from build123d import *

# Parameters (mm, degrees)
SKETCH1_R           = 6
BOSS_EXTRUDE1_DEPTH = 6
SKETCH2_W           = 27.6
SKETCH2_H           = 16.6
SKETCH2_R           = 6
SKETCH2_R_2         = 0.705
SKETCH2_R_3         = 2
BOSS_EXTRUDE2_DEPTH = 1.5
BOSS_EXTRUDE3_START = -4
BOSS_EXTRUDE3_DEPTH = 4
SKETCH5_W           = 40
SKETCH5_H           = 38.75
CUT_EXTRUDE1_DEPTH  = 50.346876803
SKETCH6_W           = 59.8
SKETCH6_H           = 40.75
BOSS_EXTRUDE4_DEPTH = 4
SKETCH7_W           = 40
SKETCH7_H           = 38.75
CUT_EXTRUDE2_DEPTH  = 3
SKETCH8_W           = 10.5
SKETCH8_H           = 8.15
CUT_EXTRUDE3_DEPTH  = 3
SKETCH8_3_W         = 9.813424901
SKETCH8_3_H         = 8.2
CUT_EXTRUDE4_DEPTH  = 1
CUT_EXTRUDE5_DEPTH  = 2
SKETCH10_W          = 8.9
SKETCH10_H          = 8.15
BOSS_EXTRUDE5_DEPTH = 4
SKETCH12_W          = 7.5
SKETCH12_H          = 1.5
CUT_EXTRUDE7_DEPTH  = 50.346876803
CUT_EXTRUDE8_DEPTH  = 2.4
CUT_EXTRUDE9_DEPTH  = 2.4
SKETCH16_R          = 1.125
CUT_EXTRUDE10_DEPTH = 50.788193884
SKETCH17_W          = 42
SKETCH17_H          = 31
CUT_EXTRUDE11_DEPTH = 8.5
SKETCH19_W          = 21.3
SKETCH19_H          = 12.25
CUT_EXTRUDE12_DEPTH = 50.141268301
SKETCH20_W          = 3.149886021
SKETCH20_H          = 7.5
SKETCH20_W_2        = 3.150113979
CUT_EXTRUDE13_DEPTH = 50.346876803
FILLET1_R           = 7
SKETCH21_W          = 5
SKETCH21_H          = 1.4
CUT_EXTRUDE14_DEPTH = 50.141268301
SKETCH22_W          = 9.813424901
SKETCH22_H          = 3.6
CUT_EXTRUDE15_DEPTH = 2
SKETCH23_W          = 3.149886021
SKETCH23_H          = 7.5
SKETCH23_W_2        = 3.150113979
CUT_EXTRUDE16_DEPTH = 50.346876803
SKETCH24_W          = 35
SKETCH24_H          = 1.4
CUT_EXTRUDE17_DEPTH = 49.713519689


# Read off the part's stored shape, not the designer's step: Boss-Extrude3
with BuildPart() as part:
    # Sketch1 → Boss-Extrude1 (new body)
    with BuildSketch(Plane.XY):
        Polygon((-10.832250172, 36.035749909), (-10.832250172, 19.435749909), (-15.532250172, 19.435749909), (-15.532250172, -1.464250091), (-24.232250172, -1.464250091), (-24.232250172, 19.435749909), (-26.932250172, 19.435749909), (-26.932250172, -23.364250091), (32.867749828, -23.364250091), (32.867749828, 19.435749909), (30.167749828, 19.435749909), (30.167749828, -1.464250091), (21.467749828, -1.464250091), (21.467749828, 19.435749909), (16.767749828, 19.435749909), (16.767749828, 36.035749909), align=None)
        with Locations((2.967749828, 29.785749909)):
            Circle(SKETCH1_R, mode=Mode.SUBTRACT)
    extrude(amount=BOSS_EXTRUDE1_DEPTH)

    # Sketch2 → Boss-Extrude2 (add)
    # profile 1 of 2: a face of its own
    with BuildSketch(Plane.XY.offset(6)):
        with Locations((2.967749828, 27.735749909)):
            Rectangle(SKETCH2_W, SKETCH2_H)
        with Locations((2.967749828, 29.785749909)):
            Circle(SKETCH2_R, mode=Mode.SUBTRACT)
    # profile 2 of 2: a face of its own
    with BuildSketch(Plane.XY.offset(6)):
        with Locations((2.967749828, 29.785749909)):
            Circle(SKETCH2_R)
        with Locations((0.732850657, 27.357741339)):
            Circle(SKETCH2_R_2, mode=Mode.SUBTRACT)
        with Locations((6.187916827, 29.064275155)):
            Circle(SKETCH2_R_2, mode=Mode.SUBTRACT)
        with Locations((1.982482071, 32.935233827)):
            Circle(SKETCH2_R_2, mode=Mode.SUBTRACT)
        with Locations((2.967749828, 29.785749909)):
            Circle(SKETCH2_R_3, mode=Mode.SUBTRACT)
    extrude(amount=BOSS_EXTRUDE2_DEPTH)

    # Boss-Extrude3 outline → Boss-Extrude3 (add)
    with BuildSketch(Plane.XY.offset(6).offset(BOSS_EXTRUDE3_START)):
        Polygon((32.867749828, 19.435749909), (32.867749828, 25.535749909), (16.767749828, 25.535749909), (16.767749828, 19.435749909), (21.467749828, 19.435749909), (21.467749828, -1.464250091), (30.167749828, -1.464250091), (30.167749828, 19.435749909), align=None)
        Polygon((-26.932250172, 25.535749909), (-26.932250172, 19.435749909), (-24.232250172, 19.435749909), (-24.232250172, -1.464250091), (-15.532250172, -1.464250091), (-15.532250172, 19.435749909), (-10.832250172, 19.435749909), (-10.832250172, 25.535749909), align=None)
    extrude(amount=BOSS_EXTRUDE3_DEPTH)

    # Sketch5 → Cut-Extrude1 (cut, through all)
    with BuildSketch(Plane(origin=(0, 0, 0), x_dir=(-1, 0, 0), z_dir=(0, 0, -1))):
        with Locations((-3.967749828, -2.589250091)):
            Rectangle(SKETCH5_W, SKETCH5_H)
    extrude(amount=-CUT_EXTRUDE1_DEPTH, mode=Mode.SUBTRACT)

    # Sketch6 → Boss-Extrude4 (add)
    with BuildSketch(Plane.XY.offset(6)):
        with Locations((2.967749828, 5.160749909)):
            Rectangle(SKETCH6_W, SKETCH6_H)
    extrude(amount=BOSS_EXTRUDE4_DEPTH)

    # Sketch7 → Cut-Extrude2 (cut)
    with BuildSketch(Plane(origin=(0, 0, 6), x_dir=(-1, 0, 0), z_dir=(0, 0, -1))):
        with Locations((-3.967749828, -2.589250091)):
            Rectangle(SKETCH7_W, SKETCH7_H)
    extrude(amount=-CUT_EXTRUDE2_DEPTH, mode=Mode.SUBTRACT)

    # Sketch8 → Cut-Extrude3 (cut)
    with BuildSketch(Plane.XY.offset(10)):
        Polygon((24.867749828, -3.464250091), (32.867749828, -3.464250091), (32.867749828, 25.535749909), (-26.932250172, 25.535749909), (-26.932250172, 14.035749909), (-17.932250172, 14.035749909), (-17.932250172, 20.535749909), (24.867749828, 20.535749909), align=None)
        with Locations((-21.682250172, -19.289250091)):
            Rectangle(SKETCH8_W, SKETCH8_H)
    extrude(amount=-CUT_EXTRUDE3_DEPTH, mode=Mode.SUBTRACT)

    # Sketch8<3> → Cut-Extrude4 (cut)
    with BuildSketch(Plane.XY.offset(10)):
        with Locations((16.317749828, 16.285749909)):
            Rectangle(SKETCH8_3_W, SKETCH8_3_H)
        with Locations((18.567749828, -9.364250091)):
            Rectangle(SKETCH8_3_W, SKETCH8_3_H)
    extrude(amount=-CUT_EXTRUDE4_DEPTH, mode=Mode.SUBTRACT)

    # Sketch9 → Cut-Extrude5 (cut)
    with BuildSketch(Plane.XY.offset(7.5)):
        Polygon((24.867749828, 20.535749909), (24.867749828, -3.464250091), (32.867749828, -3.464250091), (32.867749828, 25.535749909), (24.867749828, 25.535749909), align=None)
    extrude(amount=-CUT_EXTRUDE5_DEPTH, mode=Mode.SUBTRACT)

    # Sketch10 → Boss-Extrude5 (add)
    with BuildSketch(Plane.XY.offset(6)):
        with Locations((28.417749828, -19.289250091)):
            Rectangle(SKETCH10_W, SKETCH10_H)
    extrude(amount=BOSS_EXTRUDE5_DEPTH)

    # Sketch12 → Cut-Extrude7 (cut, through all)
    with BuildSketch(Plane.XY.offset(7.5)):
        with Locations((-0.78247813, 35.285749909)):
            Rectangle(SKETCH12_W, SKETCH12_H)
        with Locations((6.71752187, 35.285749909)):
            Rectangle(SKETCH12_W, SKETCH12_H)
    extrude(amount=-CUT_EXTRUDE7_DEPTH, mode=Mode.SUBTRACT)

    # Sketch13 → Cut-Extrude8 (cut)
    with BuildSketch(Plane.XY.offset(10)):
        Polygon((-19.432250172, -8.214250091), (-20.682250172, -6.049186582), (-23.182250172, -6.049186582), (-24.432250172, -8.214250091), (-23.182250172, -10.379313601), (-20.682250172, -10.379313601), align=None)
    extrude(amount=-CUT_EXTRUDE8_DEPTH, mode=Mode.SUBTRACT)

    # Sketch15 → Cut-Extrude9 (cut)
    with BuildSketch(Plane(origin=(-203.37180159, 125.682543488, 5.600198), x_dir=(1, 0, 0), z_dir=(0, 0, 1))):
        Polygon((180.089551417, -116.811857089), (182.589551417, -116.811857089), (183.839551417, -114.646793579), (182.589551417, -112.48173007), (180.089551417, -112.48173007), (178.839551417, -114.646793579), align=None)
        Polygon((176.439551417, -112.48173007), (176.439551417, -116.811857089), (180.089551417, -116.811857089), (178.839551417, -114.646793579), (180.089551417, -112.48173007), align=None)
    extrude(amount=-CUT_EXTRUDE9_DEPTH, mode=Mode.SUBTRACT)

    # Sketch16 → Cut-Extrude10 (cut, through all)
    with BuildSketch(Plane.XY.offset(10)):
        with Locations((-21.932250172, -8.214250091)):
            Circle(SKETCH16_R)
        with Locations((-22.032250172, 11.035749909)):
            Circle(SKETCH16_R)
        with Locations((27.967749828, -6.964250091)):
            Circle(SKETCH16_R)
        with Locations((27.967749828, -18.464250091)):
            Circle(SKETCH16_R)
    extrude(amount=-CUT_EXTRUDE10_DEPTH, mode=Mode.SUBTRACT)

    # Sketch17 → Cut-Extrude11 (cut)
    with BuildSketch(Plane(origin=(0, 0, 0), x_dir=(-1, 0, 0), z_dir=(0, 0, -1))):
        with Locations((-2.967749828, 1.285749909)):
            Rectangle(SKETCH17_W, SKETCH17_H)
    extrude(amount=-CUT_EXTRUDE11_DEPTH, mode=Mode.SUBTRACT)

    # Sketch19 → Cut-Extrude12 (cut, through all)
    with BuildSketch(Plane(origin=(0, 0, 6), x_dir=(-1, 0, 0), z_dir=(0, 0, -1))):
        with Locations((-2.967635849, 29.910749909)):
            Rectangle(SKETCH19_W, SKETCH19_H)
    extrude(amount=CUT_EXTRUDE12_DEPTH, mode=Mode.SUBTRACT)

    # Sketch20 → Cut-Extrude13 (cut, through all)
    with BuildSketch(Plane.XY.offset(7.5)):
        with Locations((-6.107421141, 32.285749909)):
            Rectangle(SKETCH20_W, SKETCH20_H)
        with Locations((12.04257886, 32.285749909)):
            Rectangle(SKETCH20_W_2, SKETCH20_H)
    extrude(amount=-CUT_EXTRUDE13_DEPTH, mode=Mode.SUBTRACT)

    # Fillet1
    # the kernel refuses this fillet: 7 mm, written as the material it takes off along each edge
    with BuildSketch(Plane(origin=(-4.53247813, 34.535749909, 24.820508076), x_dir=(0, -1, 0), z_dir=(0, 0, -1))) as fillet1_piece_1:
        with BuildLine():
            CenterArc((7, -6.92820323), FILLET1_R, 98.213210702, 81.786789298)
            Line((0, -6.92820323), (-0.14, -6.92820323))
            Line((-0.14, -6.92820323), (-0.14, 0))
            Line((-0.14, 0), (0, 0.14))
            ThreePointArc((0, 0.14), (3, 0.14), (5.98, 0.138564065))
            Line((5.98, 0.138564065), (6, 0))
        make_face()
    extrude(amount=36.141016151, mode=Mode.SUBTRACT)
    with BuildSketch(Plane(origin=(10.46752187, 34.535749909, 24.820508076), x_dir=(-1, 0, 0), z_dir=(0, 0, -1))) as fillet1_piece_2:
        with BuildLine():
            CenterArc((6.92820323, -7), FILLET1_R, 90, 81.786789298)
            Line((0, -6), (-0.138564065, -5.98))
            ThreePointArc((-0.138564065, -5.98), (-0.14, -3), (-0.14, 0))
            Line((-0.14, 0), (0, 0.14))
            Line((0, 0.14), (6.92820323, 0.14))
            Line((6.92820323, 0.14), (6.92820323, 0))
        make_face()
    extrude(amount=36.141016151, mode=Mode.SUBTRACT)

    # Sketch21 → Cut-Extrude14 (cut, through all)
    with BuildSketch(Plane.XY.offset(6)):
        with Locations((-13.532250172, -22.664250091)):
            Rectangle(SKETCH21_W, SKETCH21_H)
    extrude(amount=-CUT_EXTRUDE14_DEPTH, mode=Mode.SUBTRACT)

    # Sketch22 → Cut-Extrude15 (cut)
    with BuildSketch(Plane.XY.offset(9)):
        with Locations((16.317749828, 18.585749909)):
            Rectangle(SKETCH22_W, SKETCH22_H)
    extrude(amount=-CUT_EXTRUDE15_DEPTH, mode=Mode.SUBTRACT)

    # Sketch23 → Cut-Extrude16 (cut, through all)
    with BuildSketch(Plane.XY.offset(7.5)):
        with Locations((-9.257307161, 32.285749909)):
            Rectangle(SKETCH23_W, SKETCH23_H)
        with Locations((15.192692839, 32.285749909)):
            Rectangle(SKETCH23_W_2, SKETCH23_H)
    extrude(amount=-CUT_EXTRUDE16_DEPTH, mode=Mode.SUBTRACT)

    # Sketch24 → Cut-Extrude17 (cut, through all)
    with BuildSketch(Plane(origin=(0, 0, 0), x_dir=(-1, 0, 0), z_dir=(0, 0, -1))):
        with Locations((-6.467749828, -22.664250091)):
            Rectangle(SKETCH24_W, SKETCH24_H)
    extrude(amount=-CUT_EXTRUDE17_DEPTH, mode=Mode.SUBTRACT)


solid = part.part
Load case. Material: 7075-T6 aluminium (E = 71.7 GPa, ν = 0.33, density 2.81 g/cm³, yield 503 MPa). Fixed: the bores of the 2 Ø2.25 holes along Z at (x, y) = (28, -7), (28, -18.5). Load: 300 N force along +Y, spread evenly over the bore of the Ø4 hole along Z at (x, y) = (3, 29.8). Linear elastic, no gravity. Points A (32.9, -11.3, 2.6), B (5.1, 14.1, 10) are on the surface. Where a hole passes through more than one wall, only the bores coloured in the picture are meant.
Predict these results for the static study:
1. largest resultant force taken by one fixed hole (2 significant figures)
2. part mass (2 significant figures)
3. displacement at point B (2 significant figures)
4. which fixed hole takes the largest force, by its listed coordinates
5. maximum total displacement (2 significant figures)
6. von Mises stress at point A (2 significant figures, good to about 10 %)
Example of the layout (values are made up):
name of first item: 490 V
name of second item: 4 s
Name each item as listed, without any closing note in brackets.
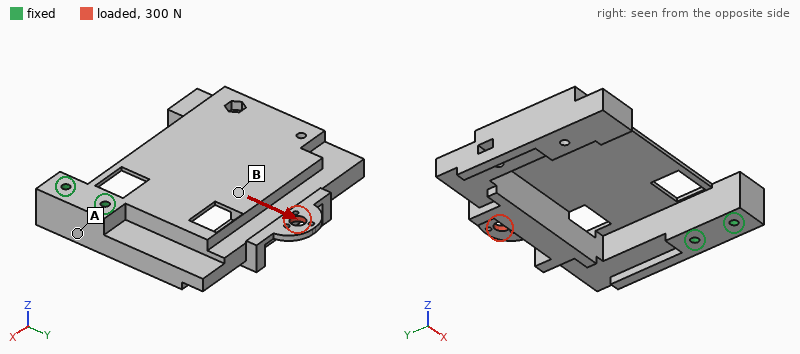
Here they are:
largest resultant force taken by one fixed hole: 560 N
part mass: 29 g
displacement at point B: 0.18 mm
which fixed hole takes the largest force, by its listed coordinates: (28, -7)
maximum total displacement: 0.43 mm
von Mises stress at point A: 21 MPa
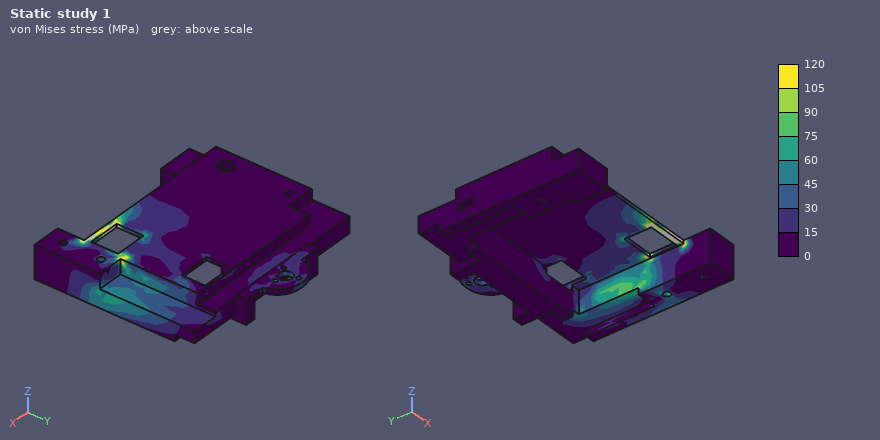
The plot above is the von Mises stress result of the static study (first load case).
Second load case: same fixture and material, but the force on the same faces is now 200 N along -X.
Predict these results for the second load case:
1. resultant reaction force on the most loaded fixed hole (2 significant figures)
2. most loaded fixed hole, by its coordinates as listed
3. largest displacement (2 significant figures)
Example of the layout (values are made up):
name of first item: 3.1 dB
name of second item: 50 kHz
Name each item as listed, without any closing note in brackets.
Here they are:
resultant reaction force on the most loaded fixed hole: 650 N
most loaded fixed hole, by its coordinates as listed: (28, -7)
largest displacement: 0.37 mm
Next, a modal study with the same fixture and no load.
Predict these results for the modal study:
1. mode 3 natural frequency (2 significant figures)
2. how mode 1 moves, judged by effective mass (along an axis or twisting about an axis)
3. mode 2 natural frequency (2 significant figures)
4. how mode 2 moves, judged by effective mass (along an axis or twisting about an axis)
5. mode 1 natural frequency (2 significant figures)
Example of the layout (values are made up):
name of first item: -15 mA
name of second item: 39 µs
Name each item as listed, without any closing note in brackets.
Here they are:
mode 3 natural frequency: 1500 Hz
how mode 1 moves, judged by effective mass: along Z
mode 2 natural frequency: 910 Hz
how mode 2 moves, judged by effective mass: along Y
mode 1 natural frequency: 370 Hz
